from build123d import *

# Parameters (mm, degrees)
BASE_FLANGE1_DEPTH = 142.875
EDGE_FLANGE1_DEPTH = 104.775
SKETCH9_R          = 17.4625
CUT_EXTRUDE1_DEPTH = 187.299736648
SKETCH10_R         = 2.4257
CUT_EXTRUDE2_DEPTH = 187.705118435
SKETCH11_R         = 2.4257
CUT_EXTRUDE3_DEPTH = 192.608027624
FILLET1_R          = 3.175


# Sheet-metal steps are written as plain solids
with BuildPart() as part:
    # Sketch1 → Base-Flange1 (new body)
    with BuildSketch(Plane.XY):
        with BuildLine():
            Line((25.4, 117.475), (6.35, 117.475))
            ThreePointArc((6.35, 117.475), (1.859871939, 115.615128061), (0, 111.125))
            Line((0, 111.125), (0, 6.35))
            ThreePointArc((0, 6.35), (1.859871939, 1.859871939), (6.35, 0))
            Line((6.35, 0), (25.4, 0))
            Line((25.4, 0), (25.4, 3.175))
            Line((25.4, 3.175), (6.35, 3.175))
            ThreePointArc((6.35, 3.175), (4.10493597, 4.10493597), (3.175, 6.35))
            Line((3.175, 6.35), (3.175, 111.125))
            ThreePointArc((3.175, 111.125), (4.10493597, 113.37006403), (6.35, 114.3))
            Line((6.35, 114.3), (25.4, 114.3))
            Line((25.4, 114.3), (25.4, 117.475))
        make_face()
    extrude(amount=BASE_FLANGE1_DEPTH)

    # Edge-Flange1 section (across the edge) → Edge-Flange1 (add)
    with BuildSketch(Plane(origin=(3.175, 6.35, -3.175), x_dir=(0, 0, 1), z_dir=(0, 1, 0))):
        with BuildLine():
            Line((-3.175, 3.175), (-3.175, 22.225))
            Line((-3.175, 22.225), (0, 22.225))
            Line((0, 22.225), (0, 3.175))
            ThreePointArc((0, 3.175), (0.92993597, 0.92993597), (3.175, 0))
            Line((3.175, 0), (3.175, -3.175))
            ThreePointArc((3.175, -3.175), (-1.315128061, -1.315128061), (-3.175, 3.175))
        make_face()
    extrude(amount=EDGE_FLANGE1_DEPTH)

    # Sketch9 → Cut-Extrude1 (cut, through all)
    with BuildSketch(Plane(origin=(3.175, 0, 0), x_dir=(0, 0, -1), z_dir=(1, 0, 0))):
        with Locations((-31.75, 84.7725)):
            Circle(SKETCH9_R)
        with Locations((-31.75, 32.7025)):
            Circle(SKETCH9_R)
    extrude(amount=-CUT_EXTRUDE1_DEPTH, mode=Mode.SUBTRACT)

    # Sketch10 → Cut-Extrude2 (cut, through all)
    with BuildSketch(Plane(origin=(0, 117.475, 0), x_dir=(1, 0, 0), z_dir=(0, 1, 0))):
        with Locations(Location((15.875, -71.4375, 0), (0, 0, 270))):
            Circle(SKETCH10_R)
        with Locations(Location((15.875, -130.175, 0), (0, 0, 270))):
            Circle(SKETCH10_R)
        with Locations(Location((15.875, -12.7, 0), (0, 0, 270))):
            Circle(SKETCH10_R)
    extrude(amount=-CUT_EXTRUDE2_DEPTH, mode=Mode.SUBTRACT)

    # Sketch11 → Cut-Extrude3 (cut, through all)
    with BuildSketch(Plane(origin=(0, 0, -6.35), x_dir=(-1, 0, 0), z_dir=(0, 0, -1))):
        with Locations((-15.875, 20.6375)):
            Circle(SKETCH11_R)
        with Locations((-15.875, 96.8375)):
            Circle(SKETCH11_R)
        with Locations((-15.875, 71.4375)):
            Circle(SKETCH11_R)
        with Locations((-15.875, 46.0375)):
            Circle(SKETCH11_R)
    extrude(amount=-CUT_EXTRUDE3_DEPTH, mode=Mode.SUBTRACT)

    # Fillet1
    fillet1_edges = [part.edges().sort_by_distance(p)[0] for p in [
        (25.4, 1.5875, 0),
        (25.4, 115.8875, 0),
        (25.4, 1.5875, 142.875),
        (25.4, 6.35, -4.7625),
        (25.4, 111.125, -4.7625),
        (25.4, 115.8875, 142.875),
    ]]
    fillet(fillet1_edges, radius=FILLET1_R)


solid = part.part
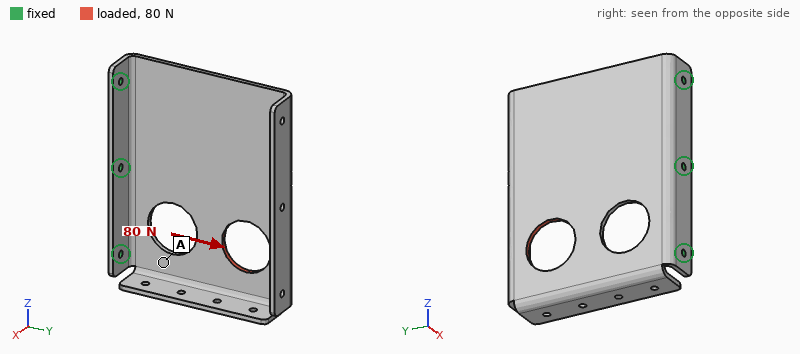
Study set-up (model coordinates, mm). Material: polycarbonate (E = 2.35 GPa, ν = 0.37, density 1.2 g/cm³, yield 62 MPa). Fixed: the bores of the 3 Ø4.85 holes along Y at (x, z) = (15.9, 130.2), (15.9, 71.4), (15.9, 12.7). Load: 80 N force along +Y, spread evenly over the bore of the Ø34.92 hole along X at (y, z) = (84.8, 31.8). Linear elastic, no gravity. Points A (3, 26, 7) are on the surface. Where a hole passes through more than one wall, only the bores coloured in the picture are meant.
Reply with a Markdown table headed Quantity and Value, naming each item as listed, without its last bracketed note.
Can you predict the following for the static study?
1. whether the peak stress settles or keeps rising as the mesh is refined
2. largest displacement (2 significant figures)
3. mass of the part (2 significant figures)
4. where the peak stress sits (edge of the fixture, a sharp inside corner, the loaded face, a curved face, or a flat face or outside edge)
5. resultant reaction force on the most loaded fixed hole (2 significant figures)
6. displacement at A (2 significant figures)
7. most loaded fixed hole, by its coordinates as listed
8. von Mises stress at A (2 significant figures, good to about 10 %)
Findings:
| Quantity | Value |
|---|---|
| whether the peak stress settles or keeps rising as the mesh is refined | keeps rising |
| largest displacement | 2.1 mm |
| mass of the part | 88 g |
| where the peak stress sits | edge of the fixture |
| resultant reaction force on the most loaded fixed hole | 53 N |
| displacement at A | 0.51 mm |
| most loaded fixed hole, by its coordinates as listed | (15.9, 12.7) |
| von Mises stress at A | 0.85 MPa |
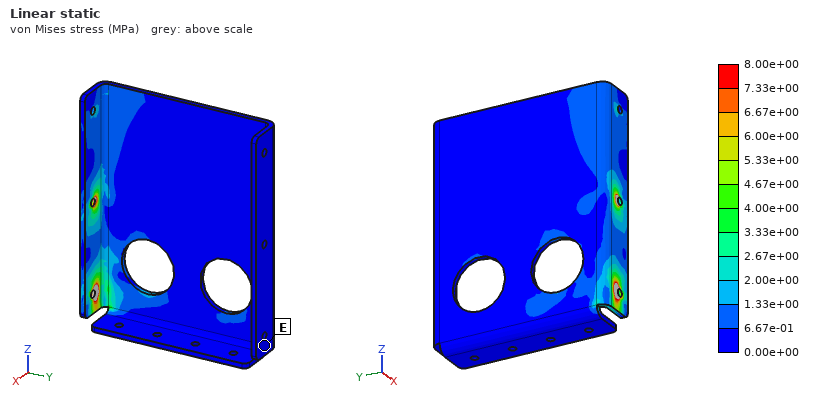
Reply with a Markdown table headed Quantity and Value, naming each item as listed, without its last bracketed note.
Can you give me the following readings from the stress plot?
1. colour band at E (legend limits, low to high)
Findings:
| Quantity | Value |
|---|---|
| colour band at E | 0.00e+00 to 6.67e-01 MPa |
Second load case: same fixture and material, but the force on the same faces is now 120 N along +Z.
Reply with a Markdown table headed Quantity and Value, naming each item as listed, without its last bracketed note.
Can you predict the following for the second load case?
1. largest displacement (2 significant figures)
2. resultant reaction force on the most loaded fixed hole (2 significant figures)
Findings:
| Quantity | Value |
|---|---|
| largest displacement | 2.2 mm |
| resultant reaction force on the most loaded fixed hole | 92 N |
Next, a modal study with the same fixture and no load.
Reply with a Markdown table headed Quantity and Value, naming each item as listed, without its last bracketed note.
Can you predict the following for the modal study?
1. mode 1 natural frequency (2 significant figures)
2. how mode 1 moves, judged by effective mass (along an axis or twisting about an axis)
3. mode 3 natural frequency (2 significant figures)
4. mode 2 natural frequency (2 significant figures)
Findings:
| Quantity | Value |
|---|---|
| mode 1 natural frequency | 36 Hz |
| how mode 1 moves, judged by effective mass | along X |
| mode 3 natural frequency | 240 Hz |
| mode 2 natural frequency | 75 Hz |
